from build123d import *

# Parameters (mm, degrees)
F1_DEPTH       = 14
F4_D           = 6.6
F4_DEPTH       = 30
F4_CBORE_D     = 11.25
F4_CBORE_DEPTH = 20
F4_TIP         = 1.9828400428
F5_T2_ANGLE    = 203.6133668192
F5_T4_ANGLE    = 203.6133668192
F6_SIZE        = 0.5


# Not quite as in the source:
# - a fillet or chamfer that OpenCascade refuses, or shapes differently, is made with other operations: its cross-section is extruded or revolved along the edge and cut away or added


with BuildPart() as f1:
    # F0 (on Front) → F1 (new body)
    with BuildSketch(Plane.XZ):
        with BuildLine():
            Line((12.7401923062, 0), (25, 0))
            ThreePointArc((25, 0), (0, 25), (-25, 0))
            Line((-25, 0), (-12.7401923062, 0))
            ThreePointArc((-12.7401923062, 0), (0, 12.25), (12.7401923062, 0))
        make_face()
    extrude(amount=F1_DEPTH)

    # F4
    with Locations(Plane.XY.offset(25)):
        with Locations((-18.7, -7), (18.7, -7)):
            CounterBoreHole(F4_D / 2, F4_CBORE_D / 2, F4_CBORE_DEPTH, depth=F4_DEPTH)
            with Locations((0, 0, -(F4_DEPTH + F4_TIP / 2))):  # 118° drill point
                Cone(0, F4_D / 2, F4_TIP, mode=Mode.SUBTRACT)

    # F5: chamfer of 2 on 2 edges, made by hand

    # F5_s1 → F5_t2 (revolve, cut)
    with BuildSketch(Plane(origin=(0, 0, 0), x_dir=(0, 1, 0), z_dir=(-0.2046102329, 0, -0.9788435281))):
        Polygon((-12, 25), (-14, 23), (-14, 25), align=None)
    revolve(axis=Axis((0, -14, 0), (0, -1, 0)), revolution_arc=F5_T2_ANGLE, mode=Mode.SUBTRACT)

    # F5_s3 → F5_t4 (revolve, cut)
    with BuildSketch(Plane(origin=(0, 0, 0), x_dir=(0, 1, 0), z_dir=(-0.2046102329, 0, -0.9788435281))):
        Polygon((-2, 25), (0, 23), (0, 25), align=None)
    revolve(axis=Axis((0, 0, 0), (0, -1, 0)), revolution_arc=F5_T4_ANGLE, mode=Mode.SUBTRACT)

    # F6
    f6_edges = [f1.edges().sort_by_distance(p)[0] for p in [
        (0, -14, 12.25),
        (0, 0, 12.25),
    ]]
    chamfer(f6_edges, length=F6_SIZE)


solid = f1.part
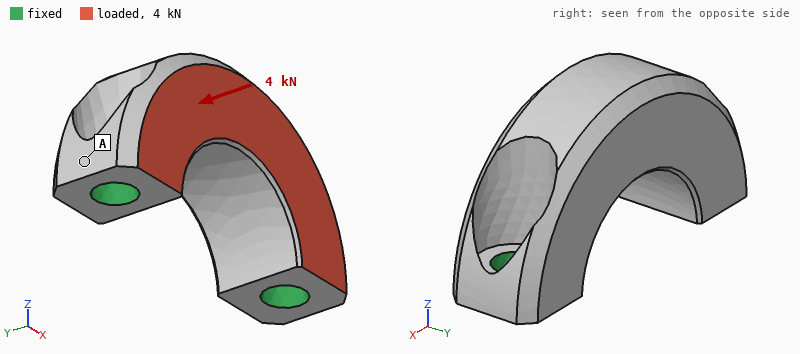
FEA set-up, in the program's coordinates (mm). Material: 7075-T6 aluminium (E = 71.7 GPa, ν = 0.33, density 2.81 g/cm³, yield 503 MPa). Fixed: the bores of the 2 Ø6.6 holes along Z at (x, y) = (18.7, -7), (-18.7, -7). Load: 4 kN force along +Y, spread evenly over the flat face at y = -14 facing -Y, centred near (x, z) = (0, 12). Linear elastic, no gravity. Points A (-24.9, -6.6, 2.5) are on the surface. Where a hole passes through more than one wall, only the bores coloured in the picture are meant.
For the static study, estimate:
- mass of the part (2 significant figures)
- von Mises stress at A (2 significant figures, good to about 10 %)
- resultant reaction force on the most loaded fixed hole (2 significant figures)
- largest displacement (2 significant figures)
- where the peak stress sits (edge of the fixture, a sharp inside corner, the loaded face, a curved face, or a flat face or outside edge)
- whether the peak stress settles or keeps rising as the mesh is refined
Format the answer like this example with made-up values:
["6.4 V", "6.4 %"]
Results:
["21 g", "32 MPa", "2.0 kN", "79 µm", "edge of the fixture", "keeps rising"]
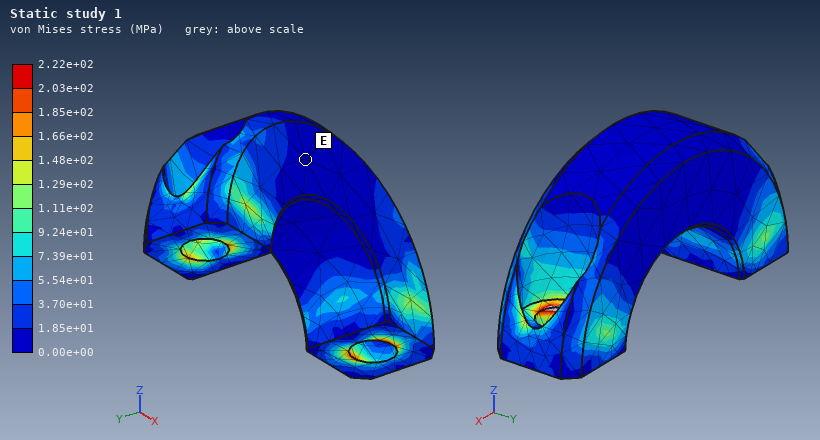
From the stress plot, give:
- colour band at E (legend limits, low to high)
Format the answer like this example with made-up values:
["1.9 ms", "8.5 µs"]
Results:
["0.00e+00 to 1.85e+01 MPa"]
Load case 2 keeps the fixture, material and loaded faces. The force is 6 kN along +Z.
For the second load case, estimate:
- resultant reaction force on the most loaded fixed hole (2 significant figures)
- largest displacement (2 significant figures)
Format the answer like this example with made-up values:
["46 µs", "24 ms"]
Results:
["3.1 kN", "74 µm"]
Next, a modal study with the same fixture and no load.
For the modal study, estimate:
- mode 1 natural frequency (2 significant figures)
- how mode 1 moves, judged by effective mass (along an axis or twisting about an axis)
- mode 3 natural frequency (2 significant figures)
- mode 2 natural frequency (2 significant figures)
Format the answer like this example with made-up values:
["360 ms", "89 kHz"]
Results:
["8600 Hz", "along Y", "20 kHz", "19 kHz"]
